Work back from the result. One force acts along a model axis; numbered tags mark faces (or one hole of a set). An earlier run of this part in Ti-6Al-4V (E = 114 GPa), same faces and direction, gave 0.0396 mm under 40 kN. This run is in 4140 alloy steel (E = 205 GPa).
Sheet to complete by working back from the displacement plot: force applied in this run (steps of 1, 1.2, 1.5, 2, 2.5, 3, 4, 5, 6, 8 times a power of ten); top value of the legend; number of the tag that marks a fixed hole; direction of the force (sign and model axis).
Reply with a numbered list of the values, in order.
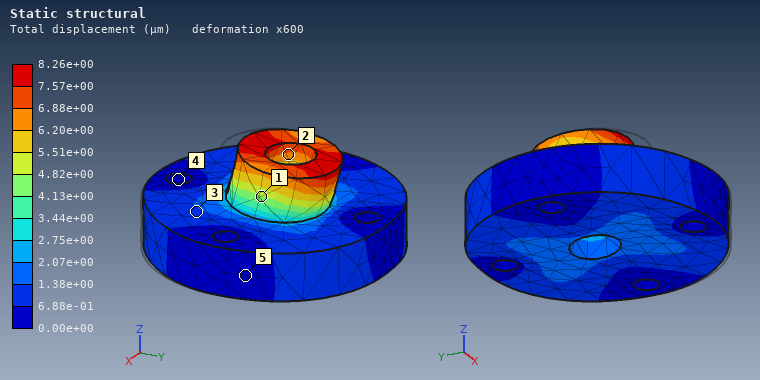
1. 15 kN
2. 8.26e+00 µm
3. 4
4. +Y
